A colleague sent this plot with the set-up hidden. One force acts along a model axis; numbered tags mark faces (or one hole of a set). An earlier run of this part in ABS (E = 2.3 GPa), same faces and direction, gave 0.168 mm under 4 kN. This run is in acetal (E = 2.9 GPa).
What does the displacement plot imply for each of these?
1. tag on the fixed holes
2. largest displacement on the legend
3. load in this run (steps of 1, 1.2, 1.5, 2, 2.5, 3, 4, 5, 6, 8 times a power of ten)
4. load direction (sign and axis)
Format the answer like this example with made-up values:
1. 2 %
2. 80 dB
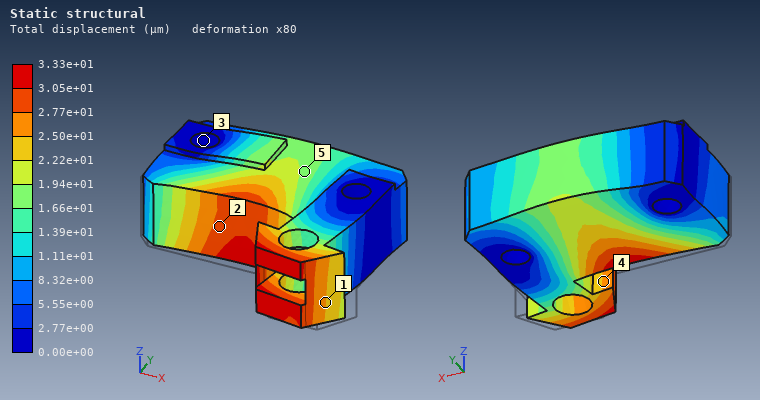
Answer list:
1. 3
2. 3.33e+01 µm
3. 1 kN
4. +Y
